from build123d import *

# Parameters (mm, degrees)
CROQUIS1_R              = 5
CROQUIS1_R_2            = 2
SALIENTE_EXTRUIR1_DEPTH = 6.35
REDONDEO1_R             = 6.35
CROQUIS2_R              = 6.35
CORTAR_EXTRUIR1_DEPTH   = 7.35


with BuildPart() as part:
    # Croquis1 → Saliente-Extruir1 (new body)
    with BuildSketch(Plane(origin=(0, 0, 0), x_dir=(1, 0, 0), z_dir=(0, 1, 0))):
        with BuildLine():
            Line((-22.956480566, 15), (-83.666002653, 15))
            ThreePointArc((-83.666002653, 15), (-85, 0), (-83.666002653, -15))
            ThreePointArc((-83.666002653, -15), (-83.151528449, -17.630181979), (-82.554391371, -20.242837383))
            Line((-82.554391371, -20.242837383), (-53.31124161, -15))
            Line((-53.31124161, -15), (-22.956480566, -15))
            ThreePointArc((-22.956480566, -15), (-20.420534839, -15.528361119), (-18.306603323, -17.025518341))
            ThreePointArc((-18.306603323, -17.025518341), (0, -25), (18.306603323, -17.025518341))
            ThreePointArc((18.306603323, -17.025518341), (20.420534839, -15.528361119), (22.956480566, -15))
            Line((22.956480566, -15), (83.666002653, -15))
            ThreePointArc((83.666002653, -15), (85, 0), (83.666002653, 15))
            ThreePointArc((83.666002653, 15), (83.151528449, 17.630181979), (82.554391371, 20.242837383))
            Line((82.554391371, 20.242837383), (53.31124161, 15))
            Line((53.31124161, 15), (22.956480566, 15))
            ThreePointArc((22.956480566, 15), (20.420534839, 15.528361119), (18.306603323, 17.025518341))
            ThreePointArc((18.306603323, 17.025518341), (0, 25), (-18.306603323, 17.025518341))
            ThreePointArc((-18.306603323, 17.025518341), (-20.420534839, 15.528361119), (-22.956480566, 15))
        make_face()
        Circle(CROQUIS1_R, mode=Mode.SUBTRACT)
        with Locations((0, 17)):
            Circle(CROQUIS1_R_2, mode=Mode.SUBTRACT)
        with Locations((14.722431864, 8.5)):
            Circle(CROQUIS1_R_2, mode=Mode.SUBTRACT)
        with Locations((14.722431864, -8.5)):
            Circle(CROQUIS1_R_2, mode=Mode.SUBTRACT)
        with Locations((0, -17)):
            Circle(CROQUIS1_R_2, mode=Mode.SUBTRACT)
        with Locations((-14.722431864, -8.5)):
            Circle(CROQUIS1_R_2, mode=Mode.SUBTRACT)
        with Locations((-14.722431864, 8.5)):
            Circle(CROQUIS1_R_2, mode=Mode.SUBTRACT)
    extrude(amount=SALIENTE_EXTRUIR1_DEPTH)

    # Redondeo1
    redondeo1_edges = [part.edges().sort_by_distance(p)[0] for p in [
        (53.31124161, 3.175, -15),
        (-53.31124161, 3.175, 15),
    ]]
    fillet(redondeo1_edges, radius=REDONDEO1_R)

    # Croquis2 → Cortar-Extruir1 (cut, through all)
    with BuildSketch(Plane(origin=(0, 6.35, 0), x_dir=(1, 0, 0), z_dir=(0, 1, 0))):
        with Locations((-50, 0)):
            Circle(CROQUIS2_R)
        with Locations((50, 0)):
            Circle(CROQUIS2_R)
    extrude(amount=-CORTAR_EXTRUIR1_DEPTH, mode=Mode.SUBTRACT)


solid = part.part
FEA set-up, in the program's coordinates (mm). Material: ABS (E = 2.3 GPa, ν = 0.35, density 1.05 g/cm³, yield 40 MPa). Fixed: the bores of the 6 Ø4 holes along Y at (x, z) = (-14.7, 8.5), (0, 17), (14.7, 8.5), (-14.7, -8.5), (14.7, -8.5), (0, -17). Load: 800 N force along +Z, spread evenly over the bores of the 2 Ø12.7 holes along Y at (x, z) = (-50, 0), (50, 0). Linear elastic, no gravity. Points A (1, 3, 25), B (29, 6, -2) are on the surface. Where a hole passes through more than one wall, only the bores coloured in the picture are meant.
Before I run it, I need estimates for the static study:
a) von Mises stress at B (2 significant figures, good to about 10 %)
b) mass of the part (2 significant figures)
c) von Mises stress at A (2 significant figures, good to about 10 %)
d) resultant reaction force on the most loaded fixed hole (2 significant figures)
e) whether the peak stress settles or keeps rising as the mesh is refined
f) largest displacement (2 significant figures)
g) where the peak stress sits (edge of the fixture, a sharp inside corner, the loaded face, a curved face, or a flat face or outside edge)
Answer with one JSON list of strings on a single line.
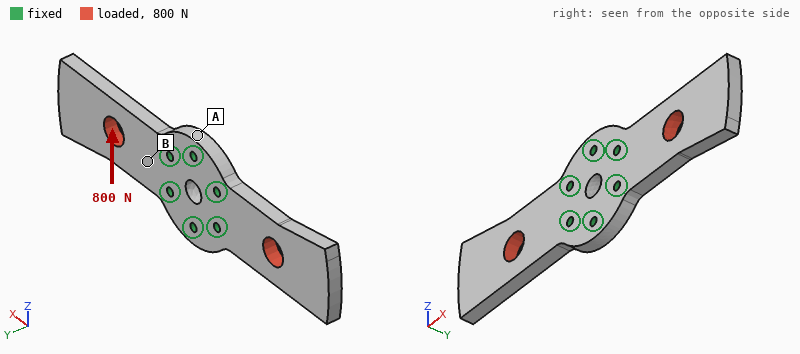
["5.7 MPa", "36 g", "1.8 MPa", "490 N", "keeps rising", "0.58 mm", "edge of the fixture"]
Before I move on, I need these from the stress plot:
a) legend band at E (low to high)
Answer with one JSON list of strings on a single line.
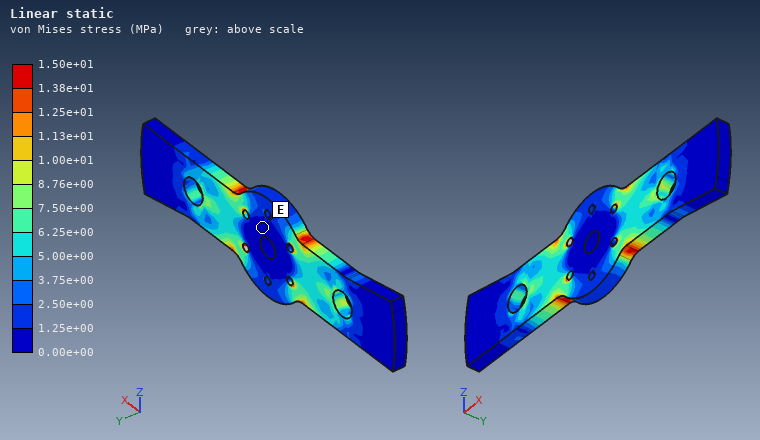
["0.00e+00 to 1.25e+00 MPa"]
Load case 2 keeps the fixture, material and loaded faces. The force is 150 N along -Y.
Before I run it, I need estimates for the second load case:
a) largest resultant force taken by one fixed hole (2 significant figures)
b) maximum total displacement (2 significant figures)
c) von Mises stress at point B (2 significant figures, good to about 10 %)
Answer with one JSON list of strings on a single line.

["60 N", "1.8 mm", "7.2 MPa"]
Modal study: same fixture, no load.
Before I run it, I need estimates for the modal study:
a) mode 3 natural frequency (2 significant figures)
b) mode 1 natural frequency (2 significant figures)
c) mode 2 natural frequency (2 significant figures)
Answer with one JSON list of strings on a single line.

["1200 Hz", "300 Hz", "300 Hz"]
